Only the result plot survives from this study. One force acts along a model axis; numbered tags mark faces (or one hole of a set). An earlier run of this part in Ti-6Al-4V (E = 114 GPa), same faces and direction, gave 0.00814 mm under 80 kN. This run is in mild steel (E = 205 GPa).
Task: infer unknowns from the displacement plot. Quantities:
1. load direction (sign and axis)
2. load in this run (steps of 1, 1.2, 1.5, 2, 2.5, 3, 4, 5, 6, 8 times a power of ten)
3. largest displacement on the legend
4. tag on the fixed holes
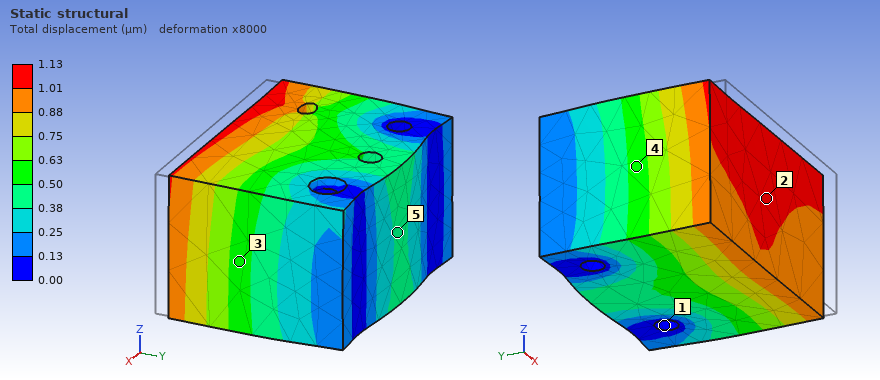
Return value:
+Y
20 kN
1.13 µm
1
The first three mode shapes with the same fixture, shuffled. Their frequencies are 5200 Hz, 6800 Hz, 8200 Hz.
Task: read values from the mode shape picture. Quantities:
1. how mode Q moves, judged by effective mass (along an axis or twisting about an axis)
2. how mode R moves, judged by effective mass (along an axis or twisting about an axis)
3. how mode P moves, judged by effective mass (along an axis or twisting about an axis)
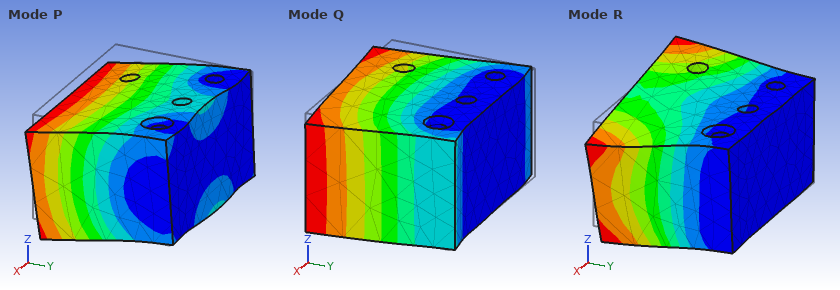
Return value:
along X
twisting about Y
along Z
